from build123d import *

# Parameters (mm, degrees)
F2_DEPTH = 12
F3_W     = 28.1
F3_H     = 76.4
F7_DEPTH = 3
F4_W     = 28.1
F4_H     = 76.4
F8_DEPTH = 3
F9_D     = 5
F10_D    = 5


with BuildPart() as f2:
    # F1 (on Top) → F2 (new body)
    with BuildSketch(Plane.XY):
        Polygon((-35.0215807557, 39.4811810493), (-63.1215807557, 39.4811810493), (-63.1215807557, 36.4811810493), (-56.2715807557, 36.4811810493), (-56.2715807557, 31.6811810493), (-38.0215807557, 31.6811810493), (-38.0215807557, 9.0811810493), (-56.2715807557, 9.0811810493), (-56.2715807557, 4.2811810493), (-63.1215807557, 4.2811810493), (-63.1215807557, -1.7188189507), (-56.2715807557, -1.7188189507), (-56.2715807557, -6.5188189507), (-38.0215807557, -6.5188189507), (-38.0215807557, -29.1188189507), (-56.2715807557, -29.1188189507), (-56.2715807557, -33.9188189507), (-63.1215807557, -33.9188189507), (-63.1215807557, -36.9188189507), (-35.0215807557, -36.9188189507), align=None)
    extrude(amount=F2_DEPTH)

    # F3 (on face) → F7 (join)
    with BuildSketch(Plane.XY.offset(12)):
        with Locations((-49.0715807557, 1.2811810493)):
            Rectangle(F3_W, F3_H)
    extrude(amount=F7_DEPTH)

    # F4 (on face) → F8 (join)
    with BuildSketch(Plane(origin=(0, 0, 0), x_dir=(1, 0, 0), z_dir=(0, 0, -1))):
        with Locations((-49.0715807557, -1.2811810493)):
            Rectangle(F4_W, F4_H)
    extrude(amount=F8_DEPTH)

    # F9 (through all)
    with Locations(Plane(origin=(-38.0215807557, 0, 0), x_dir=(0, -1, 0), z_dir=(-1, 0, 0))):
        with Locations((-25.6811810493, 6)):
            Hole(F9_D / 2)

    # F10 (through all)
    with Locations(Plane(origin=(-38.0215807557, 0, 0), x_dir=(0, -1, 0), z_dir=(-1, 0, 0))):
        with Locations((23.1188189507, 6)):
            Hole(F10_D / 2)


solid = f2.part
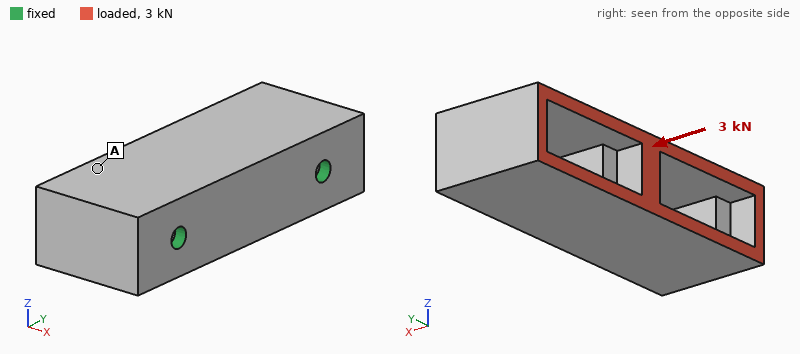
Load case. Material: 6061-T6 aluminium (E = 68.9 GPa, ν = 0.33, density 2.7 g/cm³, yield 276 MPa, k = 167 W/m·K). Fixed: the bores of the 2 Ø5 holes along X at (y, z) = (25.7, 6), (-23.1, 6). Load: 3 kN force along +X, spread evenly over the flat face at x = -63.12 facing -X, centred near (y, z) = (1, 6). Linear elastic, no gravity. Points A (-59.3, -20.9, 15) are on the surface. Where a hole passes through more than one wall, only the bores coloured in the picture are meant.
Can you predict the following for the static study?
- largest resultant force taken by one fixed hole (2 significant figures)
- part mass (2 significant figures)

1.5 kN
63 g
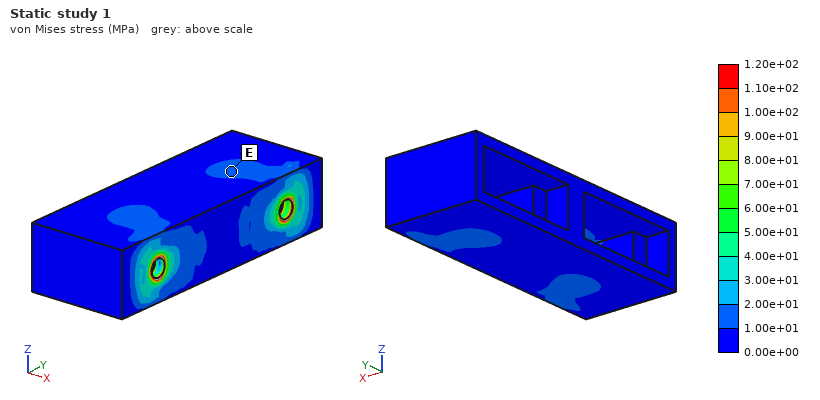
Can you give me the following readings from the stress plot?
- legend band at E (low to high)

1.00e+01 to 2.00e+01 MPa
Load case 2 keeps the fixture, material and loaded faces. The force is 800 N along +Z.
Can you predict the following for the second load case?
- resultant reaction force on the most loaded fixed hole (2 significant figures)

400 N
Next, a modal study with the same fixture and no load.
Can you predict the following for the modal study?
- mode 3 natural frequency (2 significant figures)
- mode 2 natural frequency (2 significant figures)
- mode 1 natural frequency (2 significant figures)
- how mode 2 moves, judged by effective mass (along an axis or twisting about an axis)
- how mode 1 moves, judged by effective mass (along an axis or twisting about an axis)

7800 Hz
6500 Hz
2900 Hz
twisting about X
along Z
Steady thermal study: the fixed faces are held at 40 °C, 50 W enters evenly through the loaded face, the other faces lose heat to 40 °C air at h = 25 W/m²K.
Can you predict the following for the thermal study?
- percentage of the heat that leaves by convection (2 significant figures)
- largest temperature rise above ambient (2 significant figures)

8.1 %
23 K
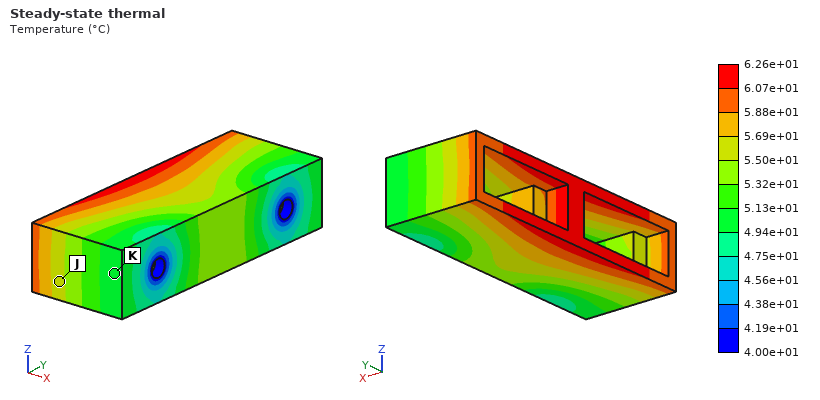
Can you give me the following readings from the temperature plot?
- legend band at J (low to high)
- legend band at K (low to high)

5.50e+01 to 5.69e+01 °C
4.94e+01 to 5.13e+01 °C
